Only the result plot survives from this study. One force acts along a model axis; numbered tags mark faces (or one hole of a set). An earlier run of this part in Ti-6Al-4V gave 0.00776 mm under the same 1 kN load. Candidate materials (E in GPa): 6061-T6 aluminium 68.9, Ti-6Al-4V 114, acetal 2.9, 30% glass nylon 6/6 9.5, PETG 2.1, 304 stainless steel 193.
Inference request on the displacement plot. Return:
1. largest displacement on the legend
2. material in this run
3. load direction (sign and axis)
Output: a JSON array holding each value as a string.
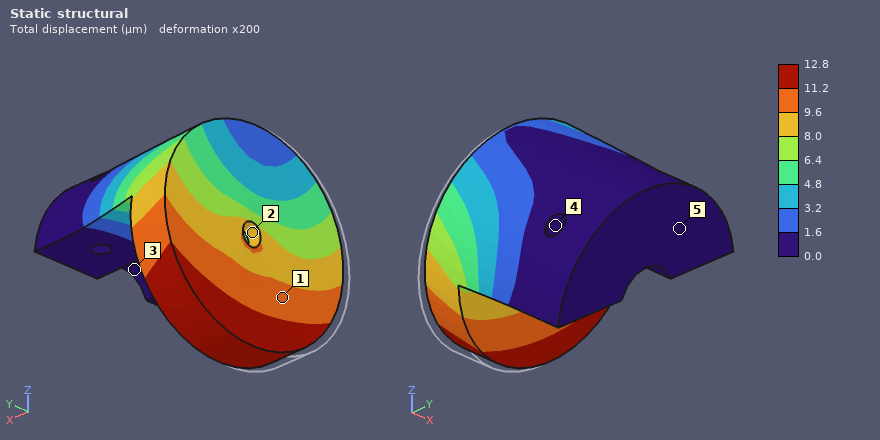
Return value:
["12.8 µm", "6061-T6 aluminium", "+Y"]
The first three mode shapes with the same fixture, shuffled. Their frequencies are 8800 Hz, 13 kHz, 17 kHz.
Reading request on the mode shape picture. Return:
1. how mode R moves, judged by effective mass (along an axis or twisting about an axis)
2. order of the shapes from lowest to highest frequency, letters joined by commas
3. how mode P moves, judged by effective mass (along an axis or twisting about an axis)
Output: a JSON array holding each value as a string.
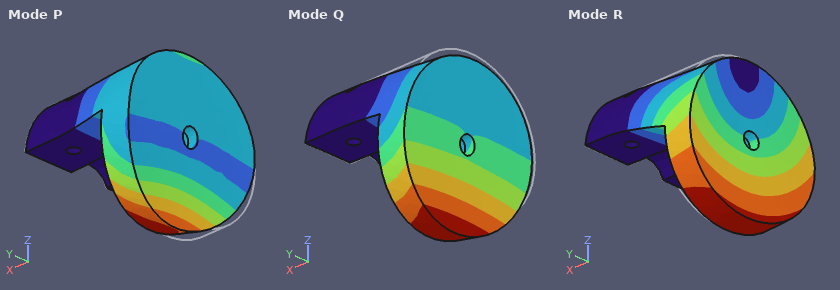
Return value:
["along Y", "Q, R, P", "along Z"]
